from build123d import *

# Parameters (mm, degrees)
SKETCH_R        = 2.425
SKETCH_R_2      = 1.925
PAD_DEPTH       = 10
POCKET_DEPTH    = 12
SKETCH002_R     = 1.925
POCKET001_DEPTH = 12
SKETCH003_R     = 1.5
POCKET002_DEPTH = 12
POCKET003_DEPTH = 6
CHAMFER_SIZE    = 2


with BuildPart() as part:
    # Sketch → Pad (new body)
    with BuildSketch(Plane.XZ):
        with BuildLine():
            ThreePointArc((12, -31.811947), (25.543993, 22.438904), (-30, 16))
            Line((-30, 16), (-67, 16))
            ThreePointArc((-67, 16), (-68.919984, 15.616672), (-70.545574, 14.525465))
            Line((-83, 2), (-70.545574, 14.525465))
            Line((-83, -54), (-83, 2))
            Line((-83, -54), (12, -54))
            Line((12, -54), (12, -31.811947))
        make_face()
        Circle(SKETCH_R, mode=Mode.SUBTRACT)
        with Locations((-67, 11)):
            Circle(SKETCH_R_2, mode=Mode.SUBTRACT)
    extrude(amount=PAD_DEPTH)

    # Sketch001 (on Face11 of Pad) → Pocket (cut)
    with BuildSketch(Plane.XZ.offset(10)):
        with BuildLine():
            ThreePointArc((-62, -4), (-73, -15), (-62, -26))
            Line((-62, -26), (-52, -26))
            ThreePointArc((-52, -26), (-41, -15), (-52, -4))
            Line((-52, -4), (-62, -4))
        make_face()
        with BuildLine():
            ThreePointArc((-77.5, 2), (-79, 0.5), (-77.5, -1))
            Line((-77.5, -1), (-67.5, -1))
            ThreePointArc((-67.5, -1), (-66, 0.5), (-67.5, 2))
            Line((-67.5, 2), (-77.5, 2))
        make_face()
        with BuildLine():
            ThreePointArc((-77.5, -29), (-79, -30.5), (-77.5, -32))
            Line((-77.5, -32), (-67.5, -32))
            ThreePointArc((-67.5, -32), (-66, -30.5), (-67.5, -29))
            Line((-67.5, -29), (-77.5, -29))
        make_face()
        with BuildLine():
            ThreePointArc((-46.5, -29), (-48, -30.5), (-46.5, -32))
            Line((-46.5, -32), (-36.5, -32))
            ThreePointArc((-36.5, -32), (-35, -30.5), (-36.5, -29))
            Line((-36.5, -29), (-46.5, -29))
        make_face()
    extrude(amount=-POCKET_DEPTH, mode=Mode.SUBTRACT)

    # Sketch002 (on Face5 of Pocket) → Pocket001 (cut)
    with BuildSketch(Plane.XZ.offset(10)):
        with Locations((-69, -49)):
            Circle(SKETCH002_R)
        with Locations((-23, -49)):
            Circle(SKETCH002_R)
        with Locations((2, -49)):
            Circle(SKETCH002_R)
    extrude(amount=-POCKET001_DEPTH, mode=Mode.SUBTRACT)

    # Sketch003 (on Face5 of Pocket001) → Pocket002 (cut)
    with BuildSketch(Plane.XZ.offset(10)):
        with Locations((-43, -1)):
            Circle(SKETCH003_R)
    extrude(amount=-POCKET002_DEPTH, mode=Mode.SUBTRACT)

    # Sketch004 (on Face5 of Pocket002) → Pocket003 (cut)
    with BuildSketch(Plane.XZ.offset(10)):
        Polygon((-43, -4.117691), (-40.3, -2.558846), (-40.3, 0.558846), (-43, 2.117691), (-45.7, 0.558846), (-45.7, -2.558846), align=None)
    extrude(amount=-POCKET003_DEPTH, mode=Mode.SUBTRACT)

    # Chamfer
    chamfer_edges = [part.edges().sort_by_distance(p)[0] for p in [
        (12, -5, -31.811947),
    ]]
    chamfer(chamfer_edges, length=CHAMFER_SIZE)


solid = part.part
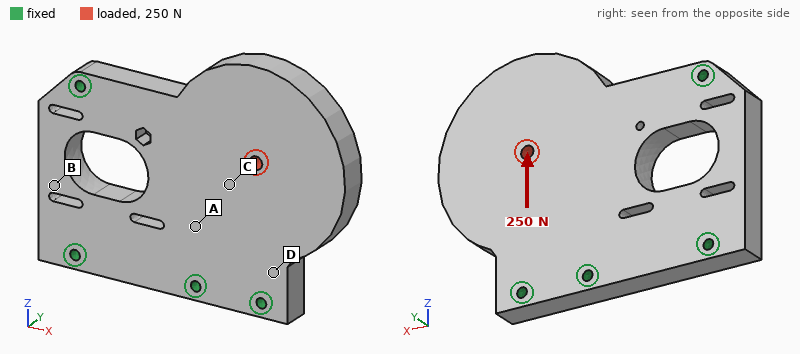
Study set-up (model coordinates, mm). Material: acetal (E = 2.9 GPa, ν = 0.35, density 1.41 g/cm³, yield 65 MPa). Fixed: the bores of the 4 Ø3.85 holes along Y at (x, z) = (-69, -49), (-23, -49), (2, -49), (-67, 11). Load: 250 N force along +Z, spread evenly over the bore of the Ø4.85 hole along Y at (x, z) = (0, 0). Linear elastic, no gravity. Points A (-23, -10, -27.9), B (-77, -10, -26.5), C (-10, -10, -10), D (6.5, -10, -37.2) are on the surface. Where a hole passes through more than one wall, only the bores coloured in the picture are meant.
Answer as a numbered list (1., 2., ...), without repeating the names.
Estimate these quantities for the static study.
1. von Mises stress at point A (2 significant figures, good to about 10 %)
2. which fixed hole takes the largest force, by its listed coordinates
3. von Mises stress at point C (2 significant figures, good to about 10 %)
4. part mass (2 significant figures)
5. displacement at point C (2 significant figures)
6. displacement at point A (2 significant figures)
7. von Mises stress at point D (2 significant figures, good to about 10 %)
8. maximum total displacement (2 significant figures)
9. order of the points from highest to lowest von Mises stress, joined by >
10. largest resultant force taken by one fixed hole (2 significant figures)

1. 0.32 MPa
2. (2, -49)
3. 0.64 MPa
4. 100 g
5. 8.3 µm
6. 3.2 µm
7. 0.88 MPa
8. 17 µm
9. D > C > A > B
10. 150 N
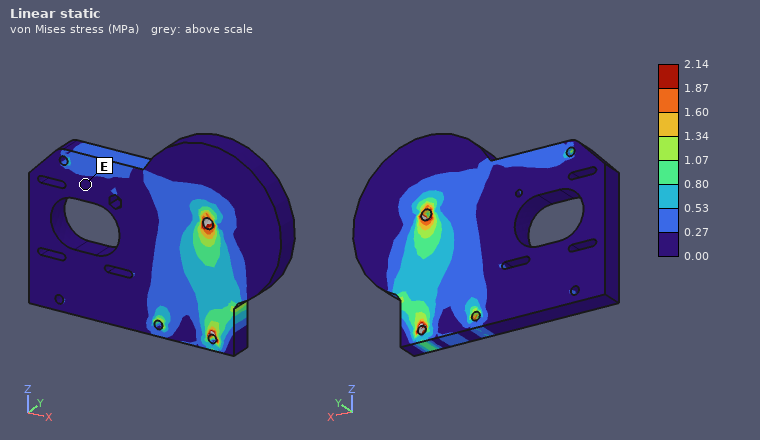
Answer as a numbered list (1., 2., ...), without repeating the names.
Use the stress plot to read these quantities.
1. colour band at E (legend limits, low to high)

1. 0.00 to 0.27 MPa
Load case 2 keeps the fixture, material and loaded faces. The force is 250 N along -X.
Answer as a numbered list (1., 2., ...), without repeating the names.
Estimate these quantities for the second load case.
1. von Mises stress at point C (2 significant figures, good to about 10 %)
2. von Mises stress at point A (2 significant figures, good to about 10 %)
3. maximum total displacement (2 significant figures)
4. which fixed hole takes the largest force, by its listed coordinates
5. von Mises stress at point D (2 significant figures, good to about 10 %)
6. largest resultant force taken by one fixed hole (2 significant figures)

1. 0.57 MPa
2. 0.33 MPa
3. 22 µm
4. (-67, 11)
5. 0.34 MPa
6. 150 N
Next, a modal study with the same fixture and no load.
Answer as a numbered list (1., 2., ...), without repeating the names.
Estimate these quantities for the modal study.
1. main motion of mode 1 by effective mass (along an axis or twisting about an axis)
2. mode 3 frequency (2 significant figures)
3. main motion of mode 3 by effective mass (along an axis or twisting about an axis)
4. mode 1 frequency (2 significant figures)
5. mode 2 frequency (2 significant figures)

1. along Y
2. 2000 Hz
3. along Y
4. 430 Hz
5. 1300 Hz
